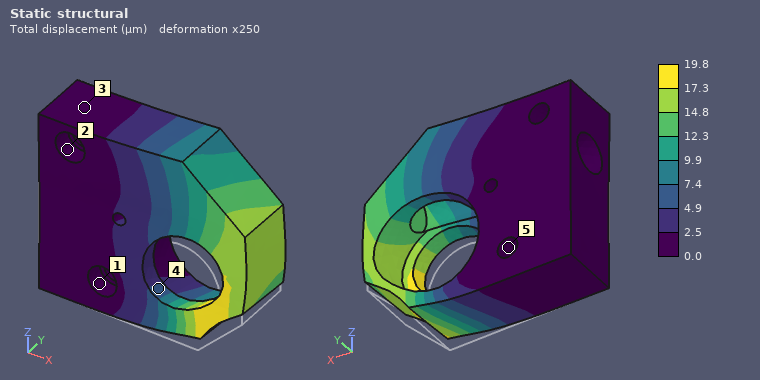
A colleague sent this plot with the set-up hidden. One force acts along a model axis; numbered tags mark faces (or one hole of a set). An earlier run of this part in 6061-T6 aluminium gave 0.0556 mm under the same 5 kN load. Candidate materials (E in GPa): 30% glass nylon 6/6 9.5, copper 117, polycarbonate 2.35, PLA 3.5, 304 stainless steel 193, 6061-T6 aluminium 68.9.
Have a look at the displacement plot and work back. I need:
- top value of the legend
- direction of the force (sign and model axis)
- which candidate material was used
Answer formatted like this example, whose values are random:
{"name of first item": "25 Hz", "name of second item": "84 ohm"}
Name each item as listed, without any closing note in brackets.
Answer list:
{"top value of the legend": "19.8 µm", "direction of the force": "+Z", "which candidate material was used": "304 stainless steel"}
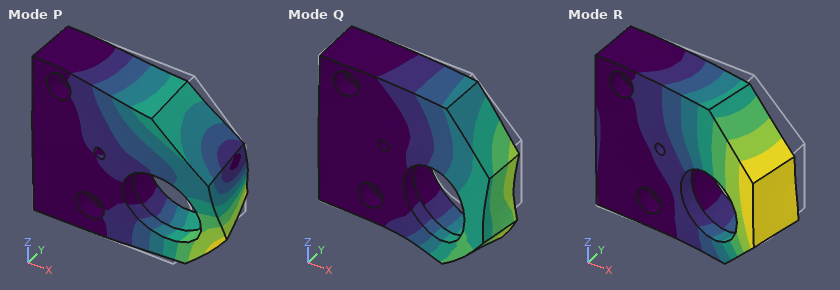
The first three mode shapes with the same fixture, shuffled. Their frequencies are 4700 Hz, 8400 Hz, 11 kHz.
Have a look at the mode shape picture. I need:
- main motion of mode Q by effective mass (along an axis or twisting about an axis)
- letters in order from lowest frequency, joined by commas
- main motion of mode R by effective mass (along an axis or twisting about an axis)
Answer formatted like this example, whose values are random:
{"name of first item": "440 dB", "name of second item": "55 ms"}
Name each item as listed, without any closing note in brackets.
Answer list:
{"main motion of mode Q by effective mass": "along Z", "letters in order from lowest frequency, joined by commas": "R, Q, P", "main motion of mode R by effective mass": "along Y"}
